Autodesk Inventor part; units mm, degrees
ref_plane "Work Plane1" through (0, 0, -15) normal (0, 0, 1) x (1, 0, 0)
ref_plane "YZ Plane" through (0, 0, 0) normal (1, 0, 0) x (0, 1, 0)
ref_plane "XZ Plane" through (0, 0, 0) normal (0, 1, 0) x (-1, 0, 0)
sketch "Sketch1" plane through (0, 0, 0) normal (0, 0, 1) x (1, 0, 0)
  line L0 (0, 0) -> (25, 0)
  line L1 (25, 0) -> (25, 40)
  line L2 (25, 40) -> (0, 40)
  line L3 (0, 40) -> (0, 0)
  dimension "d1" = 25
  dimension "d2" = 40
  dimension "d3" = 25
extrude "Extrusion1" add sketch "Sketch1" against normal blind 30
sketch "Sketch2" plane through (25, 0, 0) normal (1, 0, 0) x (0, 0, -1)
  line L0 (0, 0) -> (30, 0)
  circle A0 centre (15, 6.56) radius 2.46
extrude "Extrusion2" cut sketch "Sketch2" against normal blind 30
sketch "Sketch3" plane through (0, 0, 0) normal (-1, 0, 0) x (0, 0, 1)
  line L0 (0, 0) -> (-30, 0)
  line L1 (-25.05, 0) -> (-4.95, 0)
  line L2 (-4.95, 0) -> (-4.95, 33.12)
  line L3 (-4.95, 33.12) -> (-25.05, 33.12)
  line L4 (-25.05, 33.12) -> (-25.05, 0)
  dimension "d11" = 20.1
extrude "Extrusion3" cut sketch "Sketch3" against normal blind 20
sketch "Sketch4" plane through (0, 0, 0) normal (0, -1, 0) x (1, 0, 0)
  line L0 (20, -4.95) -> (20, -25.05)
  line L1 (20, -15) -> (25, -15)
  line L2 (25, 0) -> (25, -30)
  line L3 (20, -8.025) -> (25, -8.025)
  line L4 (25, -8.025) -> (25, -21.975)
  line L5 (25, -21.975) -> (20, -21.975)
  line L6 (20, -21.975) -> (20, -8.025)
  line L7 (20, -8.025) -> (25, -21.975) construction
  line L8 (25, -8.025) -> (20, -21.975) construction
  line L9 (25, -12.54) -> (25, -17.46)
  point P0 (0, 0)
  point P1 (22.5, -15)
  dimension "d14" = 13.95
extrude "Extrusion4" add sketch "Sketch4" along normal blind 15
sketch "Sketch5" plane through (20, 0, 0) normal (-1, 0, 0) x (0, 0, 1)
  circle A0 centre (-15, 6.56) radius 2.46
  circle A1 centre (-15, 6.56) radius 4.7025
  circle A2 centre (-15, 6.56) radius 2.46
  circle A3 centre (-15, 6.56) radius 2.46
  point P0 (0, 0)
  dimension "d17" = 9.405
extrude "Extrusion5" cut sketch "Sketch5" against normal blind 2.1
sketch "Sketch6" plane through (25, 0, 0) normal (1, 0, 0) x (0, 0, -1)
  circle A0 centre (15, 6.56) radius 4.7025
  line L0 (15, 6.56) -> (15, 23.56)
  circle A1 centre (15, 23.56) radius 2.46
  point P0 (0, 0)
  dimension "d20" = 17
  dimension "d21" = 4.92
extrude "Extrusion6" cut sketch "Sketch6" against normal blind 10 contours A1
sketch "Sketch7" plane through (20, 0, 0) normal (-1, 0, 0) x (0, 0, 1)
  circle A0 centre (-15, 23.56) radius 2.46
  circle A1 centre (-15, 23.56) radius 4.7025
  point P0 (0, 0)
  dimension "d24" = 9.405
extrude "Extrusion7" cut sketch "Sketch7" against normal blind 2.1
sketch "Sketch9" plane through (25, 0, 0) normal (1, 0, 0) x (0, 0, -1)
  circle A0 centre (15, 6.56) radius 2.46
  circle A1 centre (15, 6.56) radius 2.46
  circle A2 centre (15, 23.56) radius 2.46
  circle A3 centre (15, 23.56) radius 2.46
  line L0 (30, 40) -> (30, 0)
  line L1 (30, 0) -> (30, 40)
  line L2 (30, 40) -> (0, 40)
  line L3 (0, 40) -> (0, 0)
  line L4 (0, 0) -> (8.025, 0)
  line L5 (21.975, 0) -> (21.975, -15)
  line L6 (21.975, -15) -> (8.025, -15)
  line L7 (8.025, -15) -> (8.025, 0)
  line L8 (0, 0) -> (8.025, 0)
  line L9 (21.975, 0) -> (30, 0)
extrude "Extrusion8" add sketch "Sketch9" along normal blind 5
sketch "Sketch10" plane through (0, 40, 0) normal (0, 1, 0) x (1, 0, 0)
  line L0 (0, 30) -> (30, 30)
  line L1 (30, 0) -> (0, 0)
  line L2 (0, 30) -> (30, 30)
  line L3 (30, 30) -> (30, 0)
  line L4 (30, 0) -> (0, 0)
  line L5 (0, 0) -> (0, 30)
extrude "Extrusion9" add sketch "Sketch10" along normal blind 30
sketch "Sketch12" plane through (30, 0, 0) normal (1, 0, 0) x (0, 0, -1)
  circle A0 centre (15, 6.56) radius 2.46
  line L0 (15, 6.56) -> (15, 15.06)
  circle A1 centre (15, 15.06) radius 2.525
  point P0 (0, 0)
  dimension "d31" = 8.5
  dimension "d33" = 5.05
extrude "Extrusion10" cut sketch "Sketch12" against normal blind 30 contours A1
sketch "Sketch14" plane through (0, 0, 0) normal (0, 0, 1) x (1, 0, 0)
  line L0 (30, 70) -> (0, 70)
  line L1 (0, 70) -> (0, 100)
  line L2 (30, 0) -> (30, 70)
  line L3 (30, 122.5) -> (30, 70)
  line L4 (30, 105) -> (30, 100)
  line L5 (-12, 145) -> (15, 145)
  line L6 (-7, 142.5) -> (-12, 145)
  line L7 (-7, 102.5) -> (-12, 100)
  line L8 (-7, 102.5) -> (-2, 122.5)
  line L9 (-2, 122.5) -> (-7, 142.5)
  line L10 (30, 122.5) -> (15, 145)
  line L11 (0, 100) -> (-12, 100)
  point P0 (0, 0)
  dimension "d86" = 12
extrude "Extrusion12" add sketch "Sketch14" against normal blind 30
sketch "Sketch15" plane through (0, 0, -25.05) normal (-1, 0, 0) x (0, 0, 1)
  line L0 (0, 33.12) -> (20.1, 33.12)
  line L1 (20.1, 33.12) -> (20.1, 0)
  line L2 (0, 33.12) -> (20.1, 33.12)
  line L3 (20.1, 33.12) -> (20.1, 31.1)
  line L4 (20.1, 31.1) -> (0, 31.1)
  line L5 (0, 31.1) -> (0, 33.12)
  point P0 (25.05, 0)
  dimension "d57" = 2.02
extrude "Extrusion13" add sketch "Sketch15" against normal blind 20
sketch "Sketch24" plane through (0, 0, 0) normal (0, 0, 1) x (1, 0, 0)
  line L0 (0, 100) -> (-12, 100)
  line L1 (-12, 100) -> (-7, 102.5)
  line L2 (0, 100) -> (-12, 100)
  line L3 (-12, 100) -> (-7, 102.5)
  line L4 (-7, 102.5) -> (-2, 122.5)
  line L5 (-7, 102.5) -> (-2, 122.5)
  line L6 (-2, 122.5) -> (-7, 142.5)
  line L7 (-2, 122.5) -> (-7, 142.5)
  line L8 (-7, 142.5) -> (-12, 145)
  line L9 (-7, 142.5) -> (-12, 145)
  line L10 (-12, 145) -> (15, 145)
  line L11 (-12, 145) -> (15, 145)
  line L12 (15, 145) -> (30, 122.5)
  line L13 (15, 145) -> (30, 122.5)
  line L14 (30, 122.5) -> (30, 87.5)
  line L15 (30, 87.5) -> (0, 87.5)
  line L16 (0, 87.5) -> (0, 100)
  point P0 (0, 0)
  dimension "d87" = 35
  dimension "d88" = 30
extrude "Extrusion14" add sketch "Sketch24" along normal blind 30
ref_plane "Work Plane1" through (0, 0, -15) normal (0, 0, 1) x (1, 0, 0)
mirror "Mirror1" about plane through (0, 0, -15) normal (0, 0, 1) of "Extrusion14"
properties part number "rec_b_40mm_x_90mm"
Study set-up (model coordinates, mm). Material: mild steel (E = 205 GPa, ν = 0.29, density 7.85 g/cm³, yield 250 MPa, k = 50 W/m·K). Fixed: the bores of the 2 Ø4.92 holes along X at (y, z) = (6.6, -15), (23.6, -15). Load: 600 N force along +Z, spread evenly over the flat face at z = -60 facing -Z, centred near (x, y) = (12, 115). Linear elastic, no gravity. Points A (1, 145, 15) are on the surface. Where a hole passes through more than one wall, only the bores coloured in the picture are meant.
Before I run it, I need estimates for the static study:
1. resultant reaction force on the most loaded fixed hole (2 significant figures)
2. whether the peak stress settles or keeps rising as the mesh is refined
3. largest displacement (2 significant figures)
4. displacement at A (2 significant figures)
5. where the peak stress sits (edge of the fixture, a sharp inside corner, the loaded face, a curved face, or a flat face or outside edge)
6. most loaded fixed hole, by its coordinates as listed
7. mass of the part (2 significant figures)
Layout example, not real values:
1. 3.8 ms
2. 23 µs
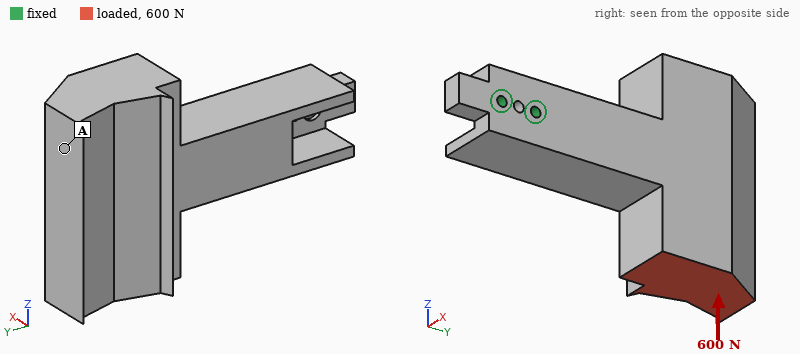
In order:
1. 2.9 kN
2. keeps rising
3. 52 µm
4. 49 µm
5. edge of the fixture
6. (23.6, -15)
7. 1.8 kg
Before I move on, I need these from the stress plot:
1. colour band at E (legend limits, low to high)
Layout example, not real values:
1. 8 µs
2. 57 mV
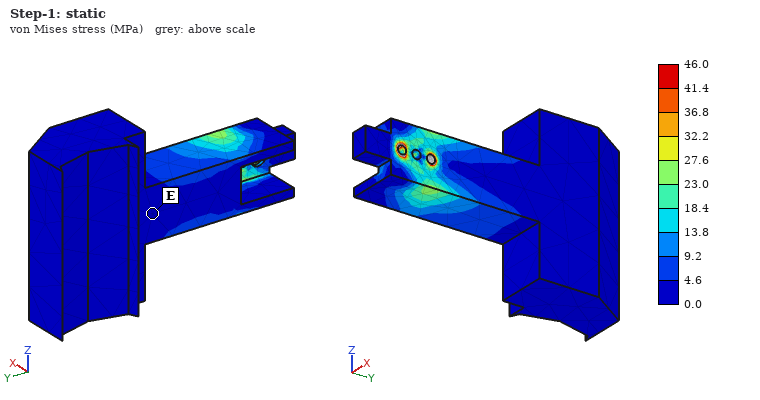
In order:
1. 0.0 to 4.6 MPa
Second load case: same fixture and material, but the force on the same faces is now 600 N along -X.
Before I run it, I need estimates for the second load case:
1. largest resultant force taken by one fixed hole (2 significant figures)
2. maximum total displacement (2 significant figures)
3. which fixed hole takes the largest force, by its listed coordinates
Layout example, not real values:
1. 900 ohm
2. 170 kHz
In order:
1. 2.8 kN
2. 95 µm
3. (23.6, -15)
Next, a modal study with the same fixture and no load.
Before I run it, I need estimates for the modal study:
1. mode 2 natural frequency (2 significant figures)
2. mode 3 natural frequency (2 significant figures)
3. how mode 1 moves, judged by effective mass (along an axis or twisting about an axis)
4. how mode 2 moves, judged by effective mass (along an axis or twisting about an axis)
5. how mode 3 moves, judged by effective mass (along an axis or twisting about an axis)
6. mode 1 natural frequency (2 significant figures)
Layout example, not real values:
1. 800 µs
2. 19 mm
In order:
1. 540 Hz
2. 1000 Hz
3. along X
4. along Z
5. twisting about Y
6. 480 Hz
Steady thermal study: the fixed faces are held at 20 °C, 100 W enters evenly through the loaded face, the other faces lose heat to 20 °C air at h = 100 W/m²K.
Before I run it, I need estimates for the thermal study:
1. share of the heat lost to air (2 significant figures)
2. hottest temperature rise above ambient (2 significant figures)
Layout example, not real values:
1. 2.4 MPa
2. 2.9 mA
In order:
1. 89 %
2. 74 K
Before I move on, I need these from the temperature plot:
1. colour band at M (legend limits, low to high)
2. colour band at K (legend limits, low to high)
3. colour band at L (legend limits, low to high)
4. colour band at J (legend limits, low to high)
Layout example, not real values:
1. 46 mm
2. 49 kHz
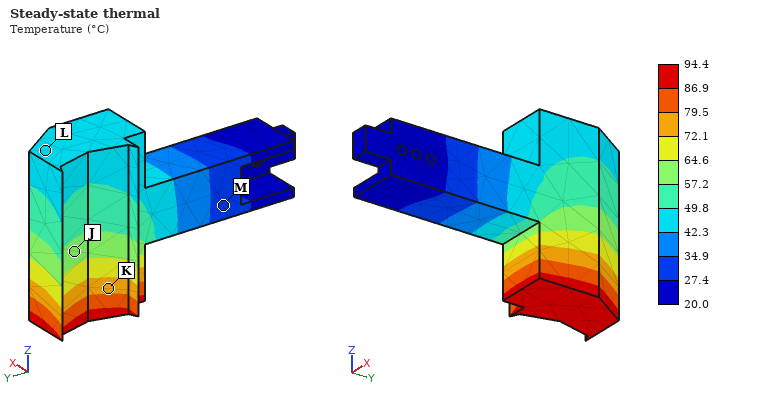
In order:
1. 27.4 to 34.9 °C
2. 72.1 to 79.5 °C
3. 42.3 to 49.8 °C
4. 57.2 to 64.6 °C
